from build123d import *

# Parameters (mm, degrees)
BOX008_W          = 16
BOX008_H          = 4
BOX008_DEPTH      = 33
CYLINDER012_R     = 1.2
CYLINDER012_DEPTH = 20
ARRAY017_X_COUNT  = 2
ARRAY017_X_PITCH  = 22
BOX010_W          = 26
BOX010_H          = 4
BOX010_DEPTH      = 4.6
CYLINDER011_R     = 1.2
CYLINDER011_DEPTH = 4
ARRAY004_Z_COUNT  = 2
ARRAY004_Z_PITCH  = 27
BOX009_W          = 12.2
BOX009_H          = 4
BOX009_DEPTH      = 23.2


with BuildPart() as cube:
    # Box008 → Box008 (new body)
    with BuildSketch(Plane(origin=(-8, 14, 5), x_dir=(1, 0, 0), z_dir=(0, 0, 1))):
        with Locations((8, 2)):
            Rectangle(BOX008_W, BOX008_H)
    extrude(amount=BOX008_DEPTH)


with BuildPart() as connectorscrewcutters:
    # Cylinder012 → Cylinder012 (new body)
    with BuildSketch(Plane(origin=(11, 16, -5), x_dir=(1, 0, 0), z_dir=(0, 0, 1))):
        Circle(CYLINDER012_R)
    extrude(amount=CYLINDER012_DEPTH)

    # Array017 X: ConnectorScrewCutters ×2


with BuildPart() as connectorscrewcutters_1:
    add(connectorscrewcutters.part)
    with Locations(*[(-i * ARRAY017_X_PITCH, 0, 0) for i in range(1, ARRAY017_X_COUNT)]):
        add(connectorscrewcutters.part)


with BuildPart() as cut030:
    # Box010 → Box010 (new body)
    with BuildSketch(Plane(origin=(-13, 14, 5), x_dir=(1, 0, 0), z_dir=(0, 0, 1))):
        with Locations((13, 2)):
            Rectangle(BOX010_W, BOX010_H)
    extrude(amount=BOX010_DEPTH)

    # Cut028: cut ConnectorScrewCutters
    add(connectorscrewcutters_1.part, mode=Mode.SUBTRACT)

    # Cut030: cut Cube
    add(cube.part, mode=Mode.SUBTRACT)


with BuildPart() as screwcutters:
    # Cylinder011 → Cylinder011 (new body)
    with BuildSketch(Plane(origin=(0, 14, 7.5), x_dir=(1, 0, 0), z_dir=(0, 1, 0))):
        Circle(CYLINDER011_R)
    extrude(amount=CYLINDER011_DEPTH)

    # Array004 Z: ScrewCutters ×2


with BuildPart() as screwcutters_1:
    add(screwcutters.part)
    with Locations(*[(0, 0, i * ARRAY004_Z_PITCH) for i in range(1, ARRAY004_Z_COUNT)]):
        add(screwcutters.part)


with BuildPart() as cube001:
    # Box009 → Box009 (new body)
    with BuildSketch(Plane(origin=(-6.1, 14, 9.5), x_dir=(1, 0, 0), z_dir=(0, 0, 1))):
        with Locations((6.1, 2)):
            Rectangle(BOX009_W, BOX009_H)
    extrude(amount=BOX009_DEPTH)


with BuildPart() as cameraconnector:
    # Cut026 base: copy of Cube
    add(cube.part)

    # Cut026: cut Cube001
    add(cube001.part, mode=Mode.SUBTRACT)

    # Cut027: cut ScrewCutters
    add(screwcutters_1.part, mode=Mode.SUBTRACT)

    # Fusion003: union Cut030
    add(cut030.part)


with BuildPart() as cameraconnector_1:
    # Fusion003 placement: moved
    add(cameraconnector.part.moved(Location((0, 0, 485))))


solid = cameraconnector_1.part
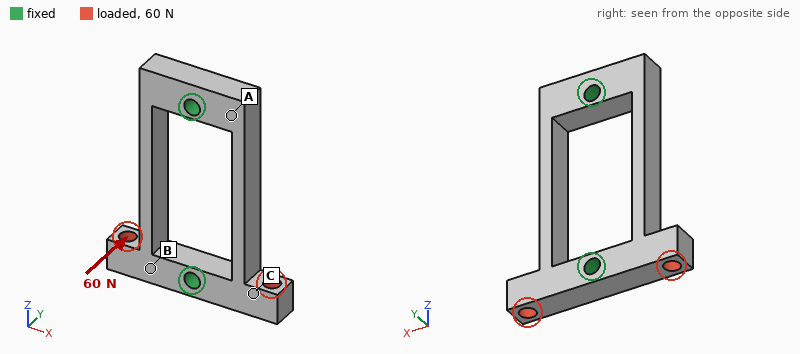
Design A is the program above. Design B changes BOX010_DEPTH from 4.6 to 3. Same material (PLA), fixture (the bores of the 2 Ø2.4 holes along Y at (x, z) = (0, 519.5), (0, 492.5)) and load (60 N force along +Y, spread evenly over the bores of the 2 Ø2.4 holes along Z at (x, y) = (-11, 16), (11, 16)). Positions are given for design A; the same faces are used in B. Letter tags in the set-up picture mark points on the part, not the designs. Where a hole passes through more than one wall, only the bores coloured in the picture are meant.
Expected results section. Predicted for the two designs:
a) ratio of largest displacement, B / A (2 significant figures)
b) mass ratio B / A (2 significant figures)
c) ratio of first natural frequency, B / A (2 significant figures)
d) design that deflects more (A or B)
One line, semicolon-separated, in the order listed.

1.1; 0.95; 0.99; B
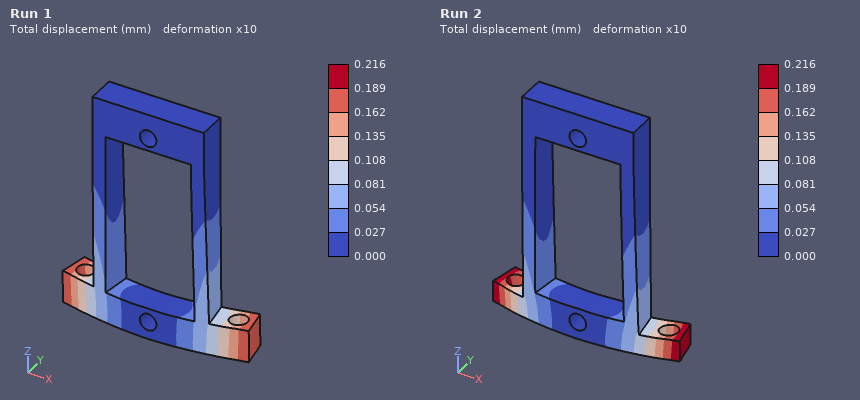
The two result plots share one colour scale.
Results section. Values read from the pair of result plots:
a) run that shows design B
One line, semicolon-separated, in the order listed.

Run 2
